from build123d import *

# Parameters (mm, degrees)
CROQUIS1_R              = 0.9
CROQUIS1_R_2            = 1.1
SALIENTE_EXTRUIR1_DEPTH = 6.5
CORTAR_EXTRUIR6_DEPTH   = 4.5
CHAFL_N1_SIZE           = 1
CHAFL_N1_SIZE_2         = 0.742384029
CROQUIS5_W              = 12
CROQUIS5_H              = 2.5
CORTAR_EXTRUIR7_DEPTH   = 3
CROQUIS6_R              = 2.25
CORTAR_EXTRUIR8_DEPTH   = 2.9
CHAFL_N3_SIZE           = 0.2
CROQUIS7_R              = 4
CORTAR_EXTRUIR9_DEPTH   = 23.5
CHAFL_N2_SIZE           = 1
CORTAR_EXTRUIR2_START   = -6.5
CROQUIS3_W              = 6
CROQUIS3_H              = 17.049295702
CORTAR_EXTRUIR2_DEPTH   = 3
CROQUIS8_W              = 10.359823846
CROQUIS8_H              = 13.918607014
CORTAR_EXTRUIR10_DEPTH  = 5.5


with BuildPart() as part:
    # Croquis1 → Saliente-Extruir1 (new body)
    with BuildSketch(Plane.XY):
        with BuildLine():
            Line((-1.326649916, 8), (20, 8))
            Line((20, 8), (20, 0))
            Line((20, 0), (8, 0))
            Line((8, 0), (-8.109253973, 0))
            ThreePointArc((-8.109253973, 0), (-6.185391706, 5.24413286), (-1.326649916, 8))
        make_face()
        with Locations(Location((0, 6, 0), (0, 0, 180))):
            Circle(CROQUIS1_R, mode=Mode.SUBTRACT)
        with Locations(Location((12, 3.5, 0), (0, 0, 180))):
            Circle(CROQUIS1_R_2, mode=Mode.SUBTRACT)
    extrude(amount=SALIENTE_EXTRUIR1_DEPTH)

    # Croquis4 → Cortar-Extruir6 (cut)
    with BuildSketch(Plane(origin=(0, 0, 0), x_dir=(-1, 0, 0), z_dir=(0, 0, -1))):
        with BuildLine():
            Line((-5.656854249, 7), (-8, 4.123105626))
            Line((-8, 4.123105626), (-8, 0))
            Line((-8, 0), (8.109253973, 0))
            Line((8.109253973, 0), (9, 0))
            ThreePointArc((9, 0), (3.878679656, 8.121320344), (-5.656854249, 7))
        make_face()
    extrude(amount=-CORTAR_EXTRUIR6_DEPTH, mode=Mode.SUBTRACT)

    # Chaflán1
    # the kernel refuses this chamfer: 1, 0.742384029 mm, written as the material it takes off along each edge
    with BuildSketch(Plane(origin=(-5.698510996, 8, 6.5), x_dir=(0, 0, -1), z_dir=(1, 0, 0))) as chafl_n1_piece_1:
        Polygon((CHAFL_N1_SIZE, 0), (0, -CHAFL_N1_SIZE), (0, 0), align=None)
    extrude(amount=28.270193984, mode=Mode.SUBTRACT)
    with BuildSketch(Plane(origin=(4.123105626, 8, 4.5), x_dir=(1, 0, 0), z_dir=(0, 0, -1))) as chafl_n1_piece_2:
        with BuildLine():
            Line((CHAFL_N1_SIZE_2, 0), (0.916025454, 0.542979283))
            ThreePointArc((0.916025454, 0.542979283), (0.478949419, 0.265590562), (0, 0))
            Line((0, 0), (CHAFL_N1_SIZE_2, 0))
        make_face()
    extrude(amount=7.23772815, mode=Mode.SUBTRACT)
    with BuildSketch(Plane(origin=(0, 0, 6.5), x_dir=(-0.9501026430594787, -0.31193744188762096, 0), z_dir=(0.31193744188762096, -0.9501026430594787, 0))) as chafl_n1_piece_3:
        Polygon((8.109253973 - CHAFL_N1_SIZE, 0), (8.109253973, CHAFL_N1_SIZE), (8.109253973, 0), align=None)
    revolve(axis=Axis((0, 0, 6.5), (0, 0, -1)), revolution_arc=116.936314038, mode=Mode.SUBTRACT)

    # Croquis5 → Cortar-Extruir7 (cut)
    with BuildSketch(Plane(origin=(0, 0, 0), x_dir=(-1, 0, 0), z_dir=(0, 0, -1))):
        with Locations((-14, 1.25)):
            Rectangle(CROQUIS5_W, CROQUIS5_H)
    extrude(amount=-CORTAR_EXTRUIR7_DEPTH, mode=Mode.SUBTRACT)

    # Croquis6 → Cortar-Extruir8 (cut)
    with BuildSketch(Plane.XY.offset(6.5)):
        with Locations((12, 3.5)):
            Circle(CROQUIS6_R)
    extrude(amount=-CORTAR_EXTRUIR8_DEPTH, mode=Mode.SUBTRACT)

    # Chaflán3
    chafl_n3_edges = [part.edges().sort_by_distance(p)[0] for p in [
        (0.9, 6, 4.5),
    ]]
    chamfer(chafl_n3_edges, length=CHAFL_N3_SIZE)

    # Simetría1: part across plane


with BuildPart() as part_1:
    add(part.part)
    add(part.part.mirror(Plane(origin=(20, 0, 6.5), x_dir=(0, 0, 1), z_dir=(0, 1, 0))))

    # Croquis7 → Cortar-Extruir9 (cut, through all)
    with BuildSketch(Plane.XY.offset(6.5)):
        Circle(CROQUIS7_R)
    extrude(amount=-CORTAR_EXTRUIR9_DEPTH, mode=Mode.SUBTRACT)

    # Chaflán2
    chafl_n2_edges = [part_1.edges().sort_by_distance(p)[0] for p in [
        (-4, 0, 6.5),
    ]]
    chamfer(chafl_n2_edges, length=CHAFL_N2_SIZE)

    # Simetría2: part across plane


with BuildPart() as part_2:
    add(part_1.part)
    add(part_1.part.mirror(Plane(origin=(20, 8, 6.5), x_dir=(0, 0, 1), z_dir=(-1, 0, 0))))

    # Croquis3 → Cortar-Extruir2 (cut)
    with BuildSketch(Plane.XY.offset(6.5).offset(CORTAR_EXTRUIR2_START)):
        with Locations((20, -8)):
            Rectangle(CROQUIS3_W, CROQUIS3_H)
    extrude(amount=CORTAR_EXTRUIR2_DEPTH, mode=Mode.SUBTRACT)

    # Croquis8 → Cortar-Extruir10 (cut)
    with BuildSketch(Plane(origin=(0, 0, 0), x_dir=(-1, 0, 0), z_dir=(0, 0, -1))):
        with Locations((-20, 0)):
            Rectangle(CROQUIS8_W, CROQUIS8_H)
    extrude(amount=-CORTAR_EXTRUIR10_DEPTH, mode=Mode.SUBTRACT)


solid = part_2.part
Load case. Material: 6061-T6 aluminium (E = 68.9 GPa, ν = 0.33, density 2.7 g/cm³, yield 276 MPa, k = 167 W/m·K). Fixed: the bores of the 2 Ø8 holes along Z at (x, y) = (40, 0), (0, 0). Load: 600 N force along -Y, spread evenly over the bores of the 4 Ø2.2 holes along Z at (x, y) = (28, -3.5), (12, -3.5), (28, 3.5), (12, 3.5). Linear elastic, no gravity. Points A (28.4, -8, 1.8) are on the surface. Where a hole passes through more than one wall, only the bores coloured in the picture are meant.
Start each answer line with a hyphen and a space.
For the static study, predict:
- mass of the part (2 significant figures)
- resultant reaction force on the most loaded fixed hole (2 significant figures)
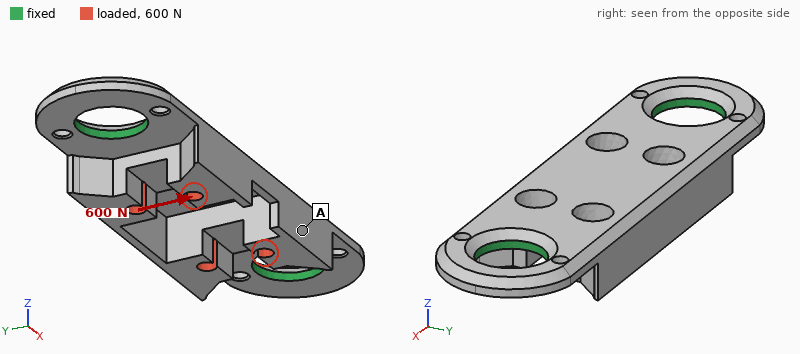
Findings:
- 5.3 g
- 300 N
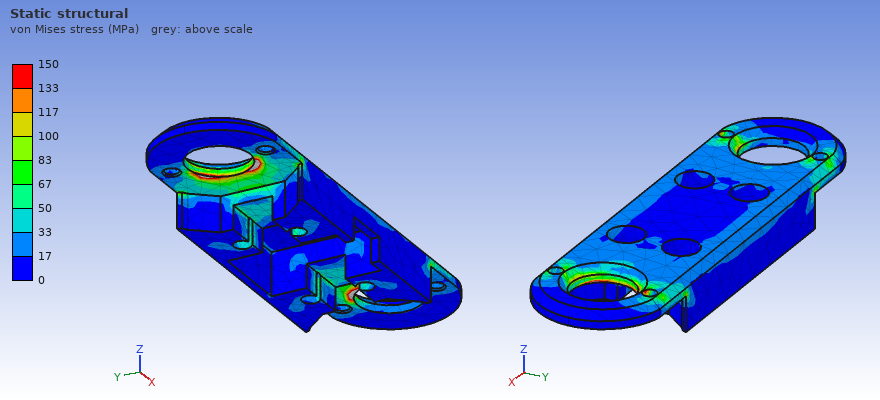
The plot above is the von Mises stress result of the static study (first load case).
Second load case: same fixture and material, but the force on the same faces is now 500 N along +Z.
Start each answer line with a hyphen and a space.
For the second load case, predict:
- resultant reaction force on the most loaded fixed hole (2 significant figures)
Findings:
- 270 N
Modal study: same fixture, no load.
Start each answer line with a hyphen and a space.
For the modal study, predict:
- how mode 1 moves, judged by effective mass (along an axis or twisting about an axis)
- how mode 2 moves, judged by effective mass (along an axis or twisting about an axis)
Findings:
- along Z
- along Z
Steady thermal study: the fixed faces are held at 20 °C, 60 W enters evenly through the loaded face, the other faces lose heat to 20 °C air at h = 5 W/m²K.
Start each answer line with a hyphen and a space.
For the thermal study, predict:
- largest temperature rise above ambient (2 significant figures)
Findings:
- 67 K
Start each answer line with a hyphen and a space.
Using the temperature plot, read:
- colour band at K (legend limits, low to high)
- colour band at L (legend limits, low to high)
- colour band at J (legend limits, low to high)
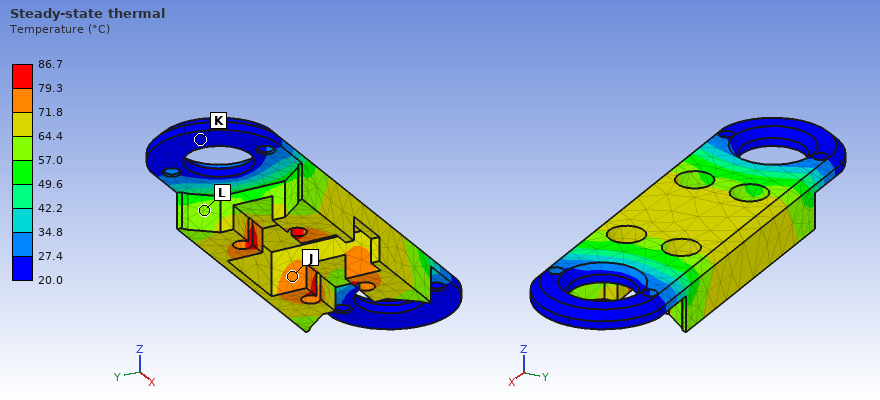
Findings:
- 20.0 to 27.4 °C
- 57.0 to 64.4 °C
- 71.8 to 79.3 °C
